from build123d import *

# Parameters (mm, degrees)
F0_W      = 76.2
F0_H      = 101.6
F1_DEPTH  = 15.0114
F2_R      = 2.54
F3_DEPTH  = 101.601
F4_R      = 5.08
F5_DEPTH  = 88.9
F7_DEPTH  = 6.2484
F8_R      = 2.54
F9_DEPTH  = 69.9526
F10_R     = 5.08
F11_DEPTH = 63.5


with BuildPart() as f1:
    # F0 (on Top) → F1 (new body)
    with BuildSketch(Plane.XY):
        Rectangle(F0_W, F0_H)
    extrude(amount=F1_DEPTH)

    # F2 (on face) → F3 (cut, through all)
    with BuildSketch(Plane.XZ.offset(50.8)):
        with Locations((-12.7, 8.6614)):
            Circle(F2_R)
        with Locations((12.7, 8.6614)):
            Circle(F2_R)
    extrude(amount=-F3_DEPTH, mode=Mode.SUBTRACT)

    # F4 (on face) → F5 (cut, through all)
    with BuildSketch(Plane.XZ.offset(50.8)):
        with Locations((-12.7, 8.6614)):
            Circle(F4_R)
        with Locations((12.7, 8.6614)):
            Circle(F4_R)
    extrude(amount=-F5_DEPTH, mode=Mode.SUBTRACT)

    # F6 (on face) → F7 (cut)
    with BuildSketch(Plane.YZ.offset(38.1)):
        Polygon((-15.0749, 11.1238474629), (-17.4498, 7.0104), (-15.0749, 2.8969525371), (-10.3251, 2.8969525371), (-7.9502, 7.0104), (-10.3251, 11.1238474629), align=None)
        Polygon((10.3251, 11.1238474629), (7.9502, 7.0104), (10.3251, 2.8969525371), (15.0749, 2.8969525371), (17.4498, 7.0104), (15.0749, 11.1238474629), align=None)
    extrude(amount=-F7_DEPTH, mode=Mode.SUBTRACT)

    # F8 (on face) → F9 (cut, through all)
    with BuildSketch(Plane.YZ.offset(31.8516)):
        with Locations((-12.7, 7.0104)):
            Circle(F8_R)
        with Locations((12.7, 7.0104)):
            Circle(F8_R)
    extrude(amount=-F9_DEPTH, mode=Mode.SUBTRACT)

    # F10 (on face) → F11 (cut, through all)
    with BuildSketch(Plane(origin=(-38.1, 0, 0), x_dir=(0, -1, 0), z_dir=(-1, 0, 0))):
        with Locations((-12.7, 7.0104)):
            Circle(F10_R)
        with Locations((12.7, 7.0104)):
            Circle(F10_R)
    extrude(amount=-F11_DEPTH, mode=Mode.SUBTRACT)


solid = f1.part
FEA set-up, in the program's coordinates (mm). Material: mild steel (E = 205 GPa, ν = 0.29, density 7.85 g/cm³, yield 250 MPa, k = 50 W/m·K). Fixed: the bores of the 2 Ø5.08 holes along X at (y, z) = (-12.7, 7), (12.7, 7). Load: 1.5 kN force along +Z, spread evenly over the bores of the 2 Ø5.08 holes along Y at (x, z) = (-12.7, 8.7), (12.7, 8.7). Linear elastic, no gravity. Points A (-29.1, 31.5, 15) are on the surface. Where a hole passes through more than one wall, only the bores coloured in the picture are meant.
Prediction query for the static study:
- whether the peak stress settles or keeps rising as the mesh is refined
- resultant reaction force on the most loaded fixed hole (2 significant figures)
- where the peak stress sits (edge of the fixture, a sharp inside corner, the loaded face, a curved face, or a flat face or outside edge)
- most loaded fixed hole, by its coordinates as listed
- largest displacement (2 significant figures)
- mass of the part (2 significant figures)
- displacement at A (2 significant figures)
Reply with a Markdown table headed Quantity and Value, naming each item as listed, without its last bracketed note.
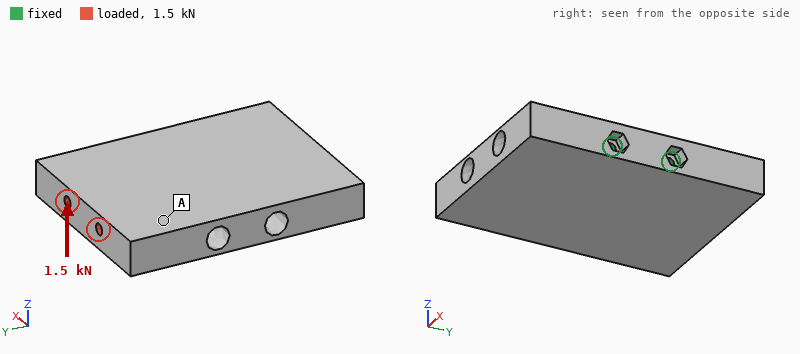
| Quantity | Value |
|---|---|
| whether the peak stress settles or keeps rising as the mesh is refined | keeps rising |
| resultant reaction force on the most loaded fixed hole | 2.8 kN |
| where the peak stress sits | edge of the fixture |
| most loaded fixed hole, by its coordinates as listed | (12.7, 7) |
| largest displacement | 77 µm |
| mass of the part | 730 g |
| displacement at A | 58 µm |
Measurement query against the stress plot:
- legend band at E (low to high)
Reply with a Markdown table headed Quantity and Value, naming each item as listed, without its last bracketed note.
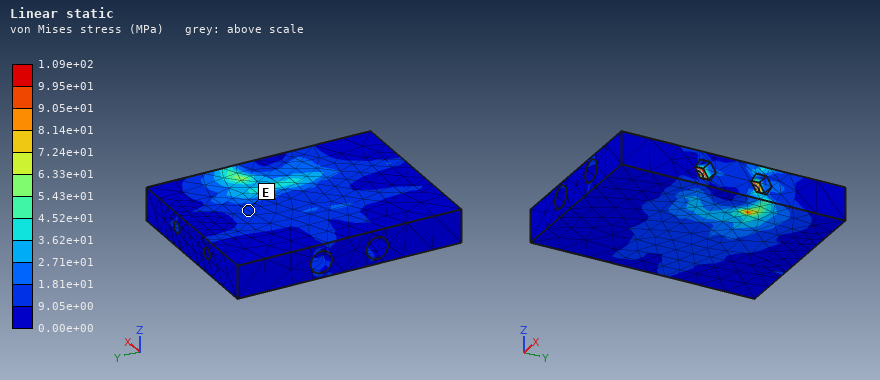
| Quantity | Value |
|---|---|
| legend band at E | 9.05e+00 to 1.81e+01 MPa |
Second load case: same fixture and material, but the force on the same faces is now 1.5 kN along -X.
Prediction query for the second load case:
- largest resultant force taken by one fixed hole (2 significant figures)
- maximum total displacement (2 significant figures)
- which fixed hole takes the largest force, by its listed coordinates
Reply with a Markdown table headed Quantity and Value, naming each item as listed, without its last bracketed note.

| Quantity | Value |
|---|---|
| largest resultant force taken by one fixed hole | 3.0 kN |
| maximum total displacement | 14 µm |
| which fixed hole takes the largest force, by its listed coordinates | (12.7, 7) |
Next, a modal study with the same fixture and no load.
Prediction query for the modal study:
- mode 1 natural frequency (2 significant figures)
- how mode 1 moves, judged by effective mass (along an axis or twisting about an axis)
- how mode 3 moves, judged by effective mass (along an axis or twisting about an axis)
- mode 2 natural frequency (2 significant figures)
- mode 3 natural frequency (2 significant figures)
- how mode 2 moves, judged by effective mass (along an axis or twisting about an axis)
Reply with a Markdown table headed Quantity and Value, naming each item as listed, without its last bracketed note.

| Quantity | Value |
|---|---|
| mode 1 natural frequency | 1200 Hz |
| how mode 1 moves, judged by effective mass | along Z |
| how mode 3 moves, judged by effective mass | along Y |
| mode 2 natural frequency | 2400 Hz |
| mode 3 natural frequency | 2600 Hz |
| how mode 2 moves, judged by effective mass | twisting about X |
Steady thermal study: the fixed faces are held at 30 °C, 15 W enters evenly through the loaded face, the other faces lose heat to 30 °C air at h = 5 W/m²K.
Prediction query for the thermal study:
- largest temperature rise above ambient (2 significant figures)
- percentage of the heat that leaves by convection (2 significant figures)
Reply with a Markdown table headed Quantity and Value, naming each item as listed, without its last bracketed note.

| Quantity | Value |
|---|---|
| largest temperature rise above ambient | 27 K |
| percentage of the heat that leaves by convection | 11 % |
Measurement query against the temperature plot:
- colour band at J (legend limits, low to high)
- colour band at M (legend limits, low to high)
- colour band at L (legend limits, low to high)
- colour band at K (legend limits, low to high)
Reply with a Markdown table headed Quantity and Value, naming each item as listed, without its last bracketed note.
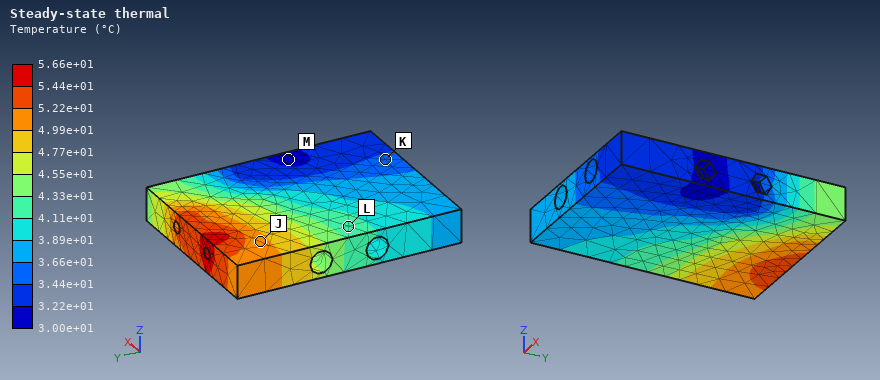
| Quantity | Value |
|---|---|
| colour band at J | 4.99e+01 to 5.22e+01 °C |
| colour band at M | 3.00e+01 to 3.22e+01 °C |
| colour band at L | 4.11e+01 to 4.33e+01 °C |
| colour band at K | 3.44e+01 to 3.66e+01 °C |
